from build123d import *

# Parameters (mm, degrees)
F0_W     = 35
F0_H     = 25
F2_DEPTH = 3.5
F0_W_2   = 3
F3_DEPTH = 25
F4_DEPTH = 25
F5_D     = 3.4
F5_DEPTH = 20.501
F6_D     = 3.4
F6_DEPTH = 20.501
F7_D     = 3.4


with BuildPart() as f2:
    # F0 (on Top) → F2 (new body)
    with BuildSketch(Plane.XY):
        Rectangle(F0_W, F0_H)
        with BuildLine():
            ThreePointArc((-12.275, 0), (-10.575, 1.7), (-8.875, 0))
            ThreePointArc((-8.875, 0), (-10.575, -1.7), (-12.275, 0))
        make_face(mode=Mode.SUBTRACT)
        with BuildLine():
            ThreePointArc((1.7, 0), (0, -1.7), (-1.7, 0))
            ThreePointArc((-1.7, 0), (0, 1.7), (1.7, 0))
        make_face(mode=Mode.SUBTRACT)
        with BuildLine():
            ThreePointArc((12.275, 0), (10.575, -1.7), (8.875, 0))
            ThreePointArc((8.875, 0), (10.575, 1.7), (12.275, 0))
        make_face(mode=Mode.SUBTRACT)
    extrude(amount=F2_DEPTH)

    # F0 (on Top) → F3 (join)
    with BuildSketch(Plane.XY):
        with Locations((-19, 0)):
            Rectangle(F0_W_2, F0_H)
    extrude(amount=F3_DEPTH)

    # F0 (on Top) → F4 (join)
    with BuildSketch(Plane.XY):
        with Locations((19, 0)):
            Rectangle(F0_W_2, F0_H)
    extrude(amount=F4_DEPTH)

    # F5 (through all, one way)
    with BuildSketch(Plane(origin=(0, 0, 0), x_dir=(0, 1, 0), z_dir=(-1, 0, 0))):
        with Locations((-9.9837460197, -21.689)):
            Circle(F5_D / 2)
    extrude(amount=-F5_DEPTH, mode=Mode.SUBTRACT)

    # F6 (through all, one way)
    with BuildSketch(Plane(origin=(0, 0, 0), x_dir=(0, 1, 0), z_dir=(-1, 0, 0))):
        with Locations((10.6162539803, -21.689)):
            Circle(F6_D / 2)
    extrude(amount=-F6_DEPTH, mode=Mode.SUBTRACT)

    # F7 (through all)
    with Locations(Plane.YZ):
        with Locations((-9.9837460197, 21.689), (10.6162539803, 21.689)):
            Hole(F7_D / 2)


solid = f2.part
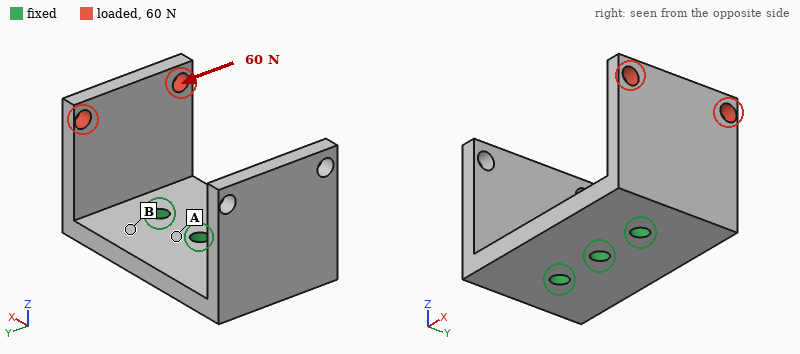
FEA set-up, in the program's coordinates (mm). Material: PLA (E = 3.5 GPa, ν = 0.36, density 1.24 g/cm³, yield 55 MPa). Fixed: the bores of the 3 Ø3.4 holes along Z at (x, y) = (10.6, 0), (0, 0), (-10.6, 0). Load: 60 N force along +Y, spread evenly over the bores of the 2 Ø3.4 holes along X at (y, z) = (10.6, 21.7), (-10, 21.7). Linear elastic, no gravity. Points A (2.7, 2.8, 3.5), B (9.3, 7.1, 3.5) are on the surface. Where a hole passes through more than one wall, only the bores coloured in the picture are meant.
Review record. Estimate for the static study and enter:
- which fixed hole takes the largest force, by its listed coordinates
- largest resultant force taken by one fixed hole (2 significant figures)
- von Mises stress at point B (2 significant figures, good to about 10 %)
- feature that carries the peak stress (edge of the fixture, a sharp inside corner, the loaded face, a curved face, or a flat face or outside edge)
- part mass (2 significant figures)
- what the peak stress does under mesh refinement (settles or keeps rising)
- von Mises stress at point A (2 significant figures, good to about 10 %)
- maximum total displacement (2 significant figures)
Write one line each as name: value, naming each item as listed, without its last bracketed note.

which fixed hole takes the largest force, by its listed coordinates: (10.6, 0)
largest resultant force taken by one fixed hole: 80 N
von Mises stress at point B: 10 MPa
feature that carries the peak stress: edge of the fixture
part mass: 8.2 g
what the peak stress does under mesh refinement: keeps rising
von Mises stress at point A: 5.0 MPa
maximum total displacement: 0.59 mm
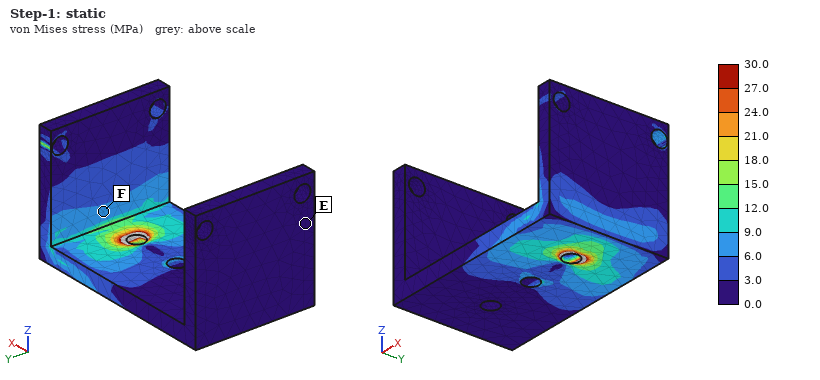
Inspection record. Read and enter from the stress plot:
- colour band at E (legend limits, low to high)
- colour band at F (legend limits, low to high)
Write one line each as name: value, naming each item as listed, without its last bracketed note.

colour band at E: 0.0 to 3.0 MPa
colour band at F: 6.0 to 9.0 MPa
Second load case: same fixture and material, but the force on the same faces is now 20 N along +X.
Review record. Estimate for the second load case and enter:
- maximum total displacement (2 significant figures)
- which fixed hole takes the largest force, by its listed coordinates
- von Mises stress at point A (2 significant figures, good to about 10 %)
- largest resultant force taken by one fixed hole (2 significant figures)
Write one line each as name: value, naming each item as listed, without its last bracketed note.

maximum total displacement: 0.55 mm
which fixed hole takes the largest force, by its listed coordinates: (10.6, 0)
von Mises stress at point A: 1.1 MPa
largest resultant force taken by one fixed hole: 23 N
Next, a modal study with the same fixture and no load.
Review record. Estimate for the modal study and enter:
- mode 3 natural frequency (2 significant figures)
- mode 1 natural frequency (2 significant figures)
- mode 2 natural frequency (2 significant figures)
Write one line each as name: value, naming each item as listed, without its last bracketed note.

mode 3 natural frequency: 1700 Hz
mode 1 natural frequency: 1200 Hz
mode 2 natural frequency: 1200 Hz
